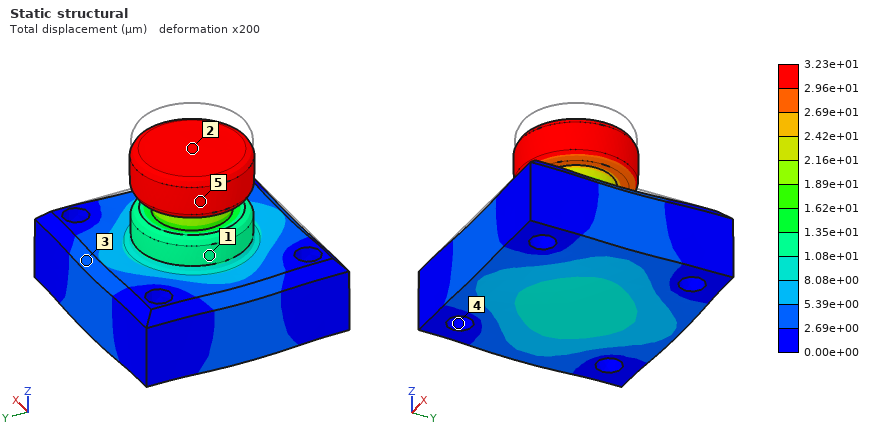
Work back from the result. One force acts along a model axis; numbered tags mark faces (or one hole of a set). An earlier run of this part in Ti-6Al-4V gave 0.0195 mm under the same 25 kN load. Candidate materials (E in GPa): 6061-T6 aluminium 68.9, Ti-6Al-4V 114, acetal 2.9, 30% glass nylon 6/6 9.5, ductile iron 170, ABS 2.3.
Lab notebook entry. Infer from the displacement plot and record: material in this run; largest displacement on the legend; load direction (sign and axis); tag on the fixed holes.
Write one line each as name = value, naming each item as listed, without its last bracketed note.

material in this run = 6061-T6 aluminium
largest displacement on the legend = 3.23e+01 µm
load direction = -Z
tag on the fixed holes = 4
